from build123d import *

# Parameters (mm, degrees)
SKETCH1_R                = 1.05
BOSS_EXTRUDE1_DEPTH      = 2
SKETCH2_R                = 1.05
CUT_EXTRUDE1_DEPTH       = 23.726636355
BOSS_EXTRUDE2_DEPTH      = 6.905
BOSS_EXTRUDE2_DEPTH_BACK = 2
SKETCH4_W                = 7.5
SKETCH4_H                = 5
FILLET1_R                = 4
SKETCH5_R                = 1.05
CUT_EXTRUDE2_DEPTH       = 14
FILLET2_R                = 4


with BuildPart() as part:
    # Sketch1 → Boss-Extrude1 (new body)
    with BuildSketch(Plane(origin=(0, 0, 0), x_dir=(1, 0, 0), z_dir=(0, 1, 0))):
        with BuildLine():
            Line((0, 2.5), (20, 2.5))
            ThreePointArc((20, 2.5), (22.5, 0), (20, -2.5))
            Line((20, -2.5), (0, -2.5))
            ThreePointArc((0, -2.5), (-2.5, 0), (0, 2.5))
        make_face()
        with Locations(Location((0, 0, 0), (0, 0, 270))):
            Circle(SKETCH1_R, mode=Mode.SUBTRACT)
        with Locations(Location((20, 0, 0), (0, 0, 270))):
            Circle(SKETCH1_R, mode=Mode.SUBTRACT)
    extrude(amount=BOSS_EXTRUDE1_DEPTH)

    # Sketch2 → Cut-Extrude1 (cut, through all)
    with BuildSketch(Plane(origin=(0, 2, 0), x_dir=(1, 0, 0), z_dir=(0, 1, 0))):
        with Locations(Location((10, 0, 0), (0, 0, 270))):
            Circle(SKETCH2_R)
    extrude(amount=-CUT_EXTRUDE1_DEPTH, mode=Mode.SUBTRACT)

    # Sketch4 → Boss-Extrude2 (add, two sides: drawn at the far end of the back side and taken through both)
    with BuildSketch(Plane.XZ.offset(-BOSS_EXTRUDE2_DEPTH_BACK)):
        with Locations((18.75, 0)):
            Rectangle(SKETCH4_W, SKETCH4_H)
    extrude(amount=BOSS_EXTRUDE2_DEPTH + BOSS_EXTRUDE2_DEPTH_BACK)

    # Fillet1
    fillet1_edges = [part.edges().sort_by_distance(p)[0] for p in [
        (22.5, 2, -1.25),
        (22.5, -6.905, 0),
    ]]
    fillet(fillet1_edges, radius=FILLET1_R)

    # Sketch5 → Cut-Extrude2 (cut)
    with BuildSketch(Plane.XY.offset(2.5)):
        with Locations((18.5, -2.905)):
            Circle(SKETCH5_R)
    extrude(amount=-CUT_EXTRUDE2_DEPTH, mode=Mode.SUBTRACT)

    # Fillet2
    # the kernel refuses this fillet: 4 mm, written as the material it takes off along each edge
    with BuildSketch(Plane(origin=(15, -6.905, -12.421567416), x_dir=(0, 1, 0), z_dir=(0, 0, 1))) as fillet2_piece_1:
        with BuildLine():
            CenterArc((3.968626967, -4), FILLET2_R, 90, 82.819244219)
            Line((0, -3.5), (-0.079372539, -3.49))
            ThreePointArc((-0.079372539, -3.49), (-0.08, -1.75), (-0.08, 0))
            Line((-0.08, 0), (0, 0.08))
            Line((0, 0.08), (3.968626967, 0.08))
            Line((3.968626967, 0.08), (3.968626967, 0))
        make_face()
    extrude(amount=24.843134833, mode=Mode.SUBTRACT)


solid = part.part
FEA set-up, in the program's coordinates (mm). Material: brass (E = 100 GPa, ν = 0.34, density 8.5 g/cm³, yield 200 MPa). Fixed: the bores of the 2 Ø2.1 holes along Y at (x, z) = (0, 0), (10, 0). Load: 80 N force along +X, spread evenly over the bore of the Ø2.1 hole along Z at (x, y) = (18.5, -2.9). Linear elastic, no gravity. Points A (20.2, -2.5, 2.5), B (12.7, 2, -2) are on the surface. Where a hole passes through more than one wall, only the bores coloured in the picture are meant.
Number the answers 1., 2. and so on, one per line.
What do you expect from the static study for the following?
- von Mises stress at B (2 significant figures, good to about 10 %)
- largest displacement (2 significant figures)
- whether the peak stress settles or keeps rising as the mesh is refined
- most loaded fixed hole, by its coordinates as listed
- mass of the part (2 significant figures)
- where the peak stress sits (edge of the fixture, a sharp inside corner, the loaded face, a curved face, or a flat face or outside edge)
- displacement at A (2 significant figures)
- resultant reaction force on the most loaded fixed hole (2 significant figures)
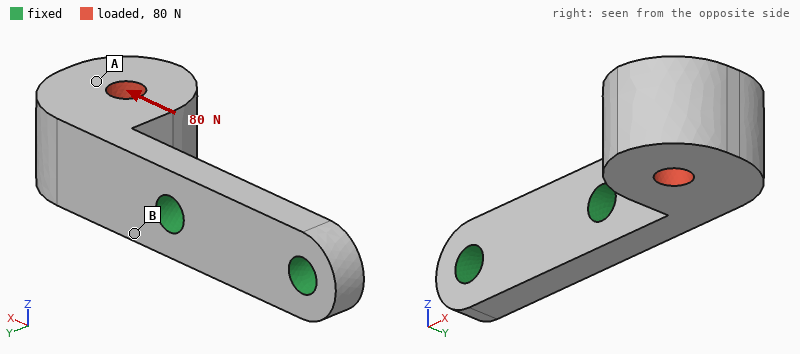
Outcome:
1. 82 MPa
2. 53 µm
3. keeps rising
4. (10, 0)
5. 3.6 g
6. edge of the fixture
7. 39 µm
8. 77 N
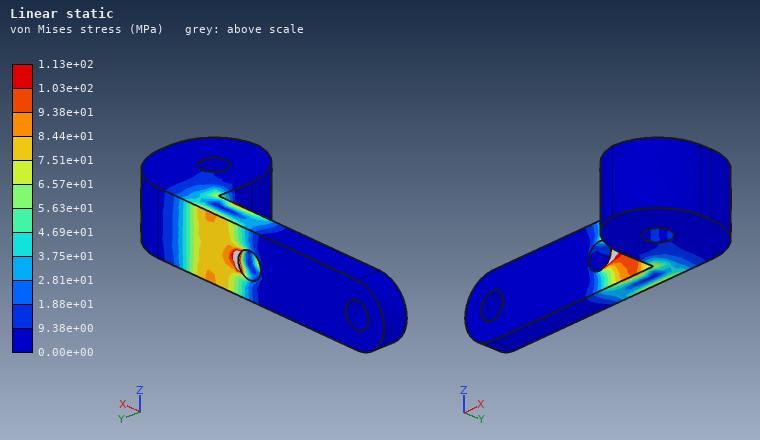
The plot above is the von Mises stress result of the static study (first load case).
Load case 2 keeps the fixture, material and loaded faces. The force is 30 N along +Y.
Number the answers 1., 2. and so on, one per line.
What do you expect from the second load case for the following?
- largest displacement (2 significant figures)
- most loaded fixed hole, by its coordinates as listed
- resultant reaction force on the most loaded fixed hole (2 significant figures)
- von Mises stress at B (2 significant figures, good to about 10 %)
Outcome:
1. 28 µm
2. (10, 0)
3. 31 N
4. 49 MPa
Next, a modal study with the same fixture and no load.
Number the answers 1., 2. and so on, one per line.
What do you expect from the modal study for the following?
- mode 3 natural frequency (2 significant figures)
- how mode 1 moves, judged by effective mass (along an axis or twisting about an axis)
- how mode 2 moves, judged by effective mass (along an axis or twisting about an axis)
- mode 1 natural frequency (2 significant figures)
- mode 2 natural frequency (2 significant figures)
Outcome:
1. 14 kHz
2. along Y
3. along Z
4. 3700 Hz
5. 6000 Hz
